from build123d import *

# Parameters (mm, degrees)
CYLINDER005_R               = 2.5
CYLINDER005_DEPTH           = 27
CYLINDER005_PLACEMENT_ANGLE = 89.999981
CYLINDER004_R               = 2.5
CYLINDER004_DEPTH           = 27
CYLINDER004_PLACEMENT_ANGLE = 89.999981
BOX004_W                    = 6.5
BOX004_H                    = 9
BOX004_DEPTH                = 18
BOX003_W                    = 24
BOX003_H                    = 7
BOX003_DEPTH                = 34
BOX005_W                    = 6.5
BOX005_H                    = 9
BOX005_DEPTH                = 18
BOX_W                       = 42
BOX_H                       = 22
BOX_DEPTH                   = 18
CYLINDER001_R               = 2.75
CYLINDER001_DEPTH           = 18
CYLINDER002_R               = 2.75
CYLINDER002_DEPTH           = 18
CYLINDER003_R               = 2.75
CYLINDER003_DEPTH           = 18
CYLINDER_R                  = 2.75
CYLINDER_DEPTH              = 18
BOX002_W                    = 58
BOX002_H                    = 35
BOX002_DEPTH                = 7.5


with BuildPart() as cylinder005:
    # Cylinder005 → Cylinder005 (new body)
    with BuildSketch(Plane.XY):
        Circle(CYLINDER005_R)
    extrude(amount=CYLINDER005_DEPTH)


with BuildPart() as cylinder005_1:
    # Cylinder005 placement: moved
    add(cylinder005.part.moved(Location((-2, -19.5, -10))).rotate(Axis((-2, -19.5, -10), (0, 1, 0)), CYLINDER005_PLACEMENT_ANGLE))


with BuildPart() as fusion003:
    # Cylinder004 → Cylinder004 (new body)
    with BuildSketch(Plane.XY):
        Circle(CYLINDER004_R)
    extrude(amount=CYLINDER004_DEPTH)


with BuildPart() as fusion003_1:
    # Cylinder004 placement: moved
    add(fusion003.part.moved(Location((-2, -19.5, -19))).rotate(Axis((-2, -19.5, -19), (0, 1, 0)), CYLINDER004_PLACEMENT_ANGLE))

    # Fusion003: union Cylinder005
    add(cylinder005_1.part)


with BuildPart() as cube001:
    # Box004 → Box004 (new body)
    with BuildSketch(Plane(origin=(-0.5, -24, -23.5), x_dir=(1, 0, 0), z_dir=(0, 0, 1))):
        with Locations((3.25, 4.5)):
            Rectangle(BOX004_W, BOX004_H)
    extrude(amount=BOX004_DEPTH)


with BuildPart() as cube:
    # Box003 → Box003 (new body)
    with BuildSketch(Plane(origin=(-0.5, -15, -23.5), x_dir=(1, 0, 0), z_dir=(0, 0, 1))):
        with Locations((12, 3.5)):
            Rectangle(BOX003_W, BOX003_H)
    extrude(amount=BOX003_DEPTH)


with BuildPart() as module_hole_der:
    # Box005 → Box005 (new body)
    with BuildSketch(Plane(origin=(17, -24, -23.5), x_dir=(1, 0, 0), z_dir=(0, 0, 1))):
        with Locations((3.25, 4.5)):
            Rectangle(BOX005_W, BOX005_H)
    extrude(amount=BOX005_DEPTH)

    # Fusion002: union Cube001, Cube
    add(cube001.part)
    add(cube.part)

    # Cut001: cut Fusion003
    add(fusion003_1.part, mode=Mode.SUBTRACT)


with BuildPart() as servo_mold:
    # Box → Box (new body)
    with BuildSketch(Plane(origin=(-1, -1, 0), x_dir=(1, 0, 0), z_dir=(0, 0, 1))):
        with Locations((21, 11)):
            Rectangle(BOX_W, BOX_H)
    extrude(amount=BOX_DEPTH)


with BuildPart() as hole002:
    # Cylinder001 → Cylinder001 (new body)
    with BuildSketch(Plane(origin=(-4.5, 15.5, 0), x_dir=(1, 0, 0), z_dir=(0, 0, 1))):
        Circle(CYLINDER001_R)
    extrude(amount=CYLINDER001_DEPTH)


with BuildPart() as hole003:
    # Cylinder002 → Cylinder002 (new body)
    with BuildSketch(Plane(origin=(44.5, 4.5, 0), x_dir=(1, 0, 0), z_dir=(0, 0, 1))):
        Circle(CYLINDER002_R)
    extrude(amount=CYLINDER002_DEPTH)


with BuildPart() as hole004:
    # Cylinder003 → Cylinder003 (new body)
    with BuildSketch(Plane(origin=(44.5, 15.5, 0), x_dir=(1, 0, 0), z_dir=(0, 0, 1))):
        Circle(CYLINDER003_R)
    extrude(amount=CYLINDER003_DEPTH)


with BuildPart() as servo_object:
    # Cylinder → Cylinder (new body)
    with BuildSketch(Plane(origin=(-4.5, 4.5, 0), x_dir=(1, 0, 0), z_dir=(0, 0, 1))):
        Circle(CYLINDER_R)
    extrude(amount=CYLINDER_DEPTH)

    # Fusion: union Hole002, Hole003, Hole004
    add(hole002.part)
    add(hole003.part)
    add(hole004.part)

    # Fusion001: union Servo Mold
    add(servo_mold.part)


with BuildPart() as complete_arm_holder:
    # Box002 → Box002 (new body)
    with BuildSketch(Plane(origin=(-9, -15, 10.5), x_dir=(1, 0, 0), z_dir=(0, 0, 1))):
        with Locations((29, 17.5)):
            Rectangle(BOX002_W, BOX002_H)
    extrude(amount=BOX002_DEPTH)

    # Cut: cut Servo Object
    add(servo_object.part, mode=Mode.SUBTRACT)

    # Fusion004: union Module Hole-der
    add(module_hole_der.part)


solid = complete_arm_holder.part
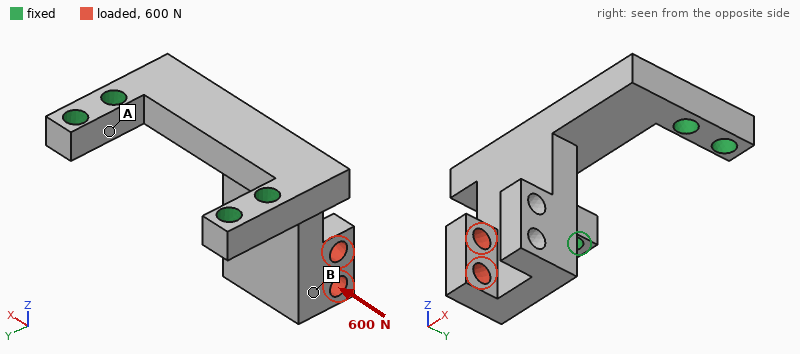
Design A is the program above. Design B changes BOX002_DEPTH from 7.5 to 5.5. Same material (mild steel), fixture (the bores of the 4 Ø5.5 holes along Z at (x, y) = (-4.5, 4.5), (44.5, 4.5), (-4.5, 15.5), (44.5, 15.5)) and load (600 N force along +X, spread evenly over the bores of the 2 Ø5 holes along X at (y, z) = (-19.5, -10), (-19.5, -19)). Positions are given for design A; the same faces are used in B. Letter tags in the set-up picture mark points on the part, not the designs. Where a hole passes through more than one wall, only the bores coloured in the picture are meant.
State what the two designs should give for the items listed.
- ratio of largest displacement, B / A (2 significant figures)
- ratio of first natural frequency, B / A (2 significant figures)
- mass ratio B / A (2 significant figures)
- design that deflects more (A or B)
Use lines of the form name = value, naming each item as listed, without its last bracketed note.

ratio of largest displacement, B / A = 1.5
ratio of first natural frequency, B / A = 0.74
mass ratio B / A = 0.86
design that deflects more = B
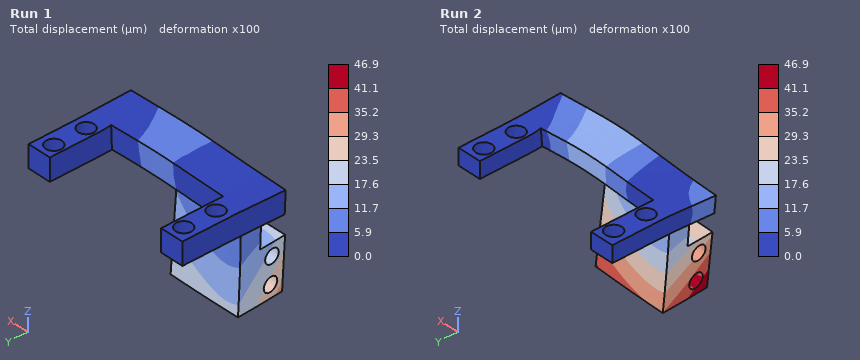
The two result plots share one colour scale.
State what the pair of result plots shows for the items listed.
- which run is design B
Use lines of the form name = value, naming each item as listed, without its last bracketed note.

which run is design B = Run 2
